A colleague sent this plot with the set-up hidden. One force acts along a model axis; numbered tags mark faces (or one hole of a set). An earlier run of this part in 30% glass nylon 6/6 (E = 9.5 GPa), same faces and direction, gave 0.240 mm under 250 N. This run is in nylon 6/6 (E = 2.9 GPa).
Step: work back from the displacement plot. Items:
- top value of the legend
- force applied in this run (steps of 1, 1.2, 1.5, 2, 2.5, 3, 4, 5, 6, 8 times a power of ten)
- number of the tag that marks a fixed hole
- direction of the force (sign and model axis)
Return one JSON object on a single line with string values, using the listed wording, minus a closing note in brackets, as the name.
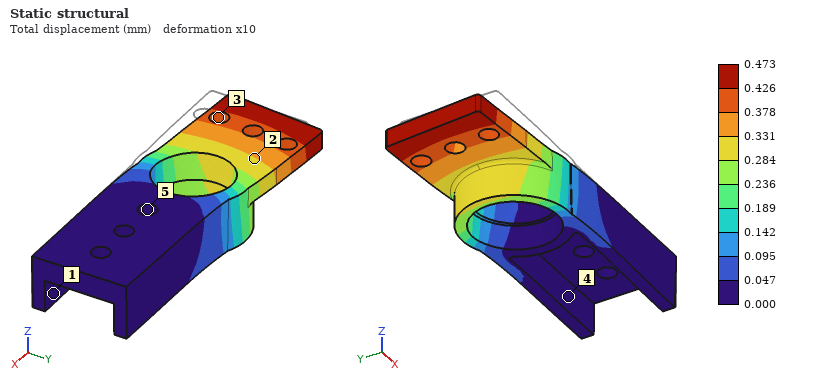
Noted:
{"top value of the legend": "0.473 mm", "force applied in this run": "150 N", "number of the tag that marks a fixed hole": "5", "direction of the force": "+Y"}
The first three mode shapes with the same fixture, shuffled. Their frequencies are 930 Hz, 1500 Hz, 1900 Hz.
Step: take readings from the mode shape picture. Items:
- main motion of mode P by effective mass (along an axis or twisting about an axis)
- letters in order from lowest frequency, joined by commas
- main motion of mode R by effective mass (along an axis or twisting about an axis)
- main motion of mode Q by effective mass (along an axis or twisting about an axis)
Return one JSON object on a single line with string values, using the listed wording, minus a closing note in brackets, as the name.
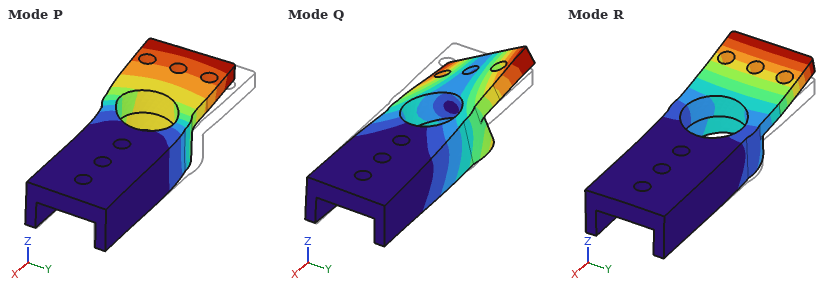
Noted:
{"main motion of mode P by effective mass": "along Y", "letters in order from lowest frequency, joined by commas": "R, P, Q", "main motion of mode R by effective mass": "along Z", "main motion of mode Q by effective mass": "twisting about X"}
